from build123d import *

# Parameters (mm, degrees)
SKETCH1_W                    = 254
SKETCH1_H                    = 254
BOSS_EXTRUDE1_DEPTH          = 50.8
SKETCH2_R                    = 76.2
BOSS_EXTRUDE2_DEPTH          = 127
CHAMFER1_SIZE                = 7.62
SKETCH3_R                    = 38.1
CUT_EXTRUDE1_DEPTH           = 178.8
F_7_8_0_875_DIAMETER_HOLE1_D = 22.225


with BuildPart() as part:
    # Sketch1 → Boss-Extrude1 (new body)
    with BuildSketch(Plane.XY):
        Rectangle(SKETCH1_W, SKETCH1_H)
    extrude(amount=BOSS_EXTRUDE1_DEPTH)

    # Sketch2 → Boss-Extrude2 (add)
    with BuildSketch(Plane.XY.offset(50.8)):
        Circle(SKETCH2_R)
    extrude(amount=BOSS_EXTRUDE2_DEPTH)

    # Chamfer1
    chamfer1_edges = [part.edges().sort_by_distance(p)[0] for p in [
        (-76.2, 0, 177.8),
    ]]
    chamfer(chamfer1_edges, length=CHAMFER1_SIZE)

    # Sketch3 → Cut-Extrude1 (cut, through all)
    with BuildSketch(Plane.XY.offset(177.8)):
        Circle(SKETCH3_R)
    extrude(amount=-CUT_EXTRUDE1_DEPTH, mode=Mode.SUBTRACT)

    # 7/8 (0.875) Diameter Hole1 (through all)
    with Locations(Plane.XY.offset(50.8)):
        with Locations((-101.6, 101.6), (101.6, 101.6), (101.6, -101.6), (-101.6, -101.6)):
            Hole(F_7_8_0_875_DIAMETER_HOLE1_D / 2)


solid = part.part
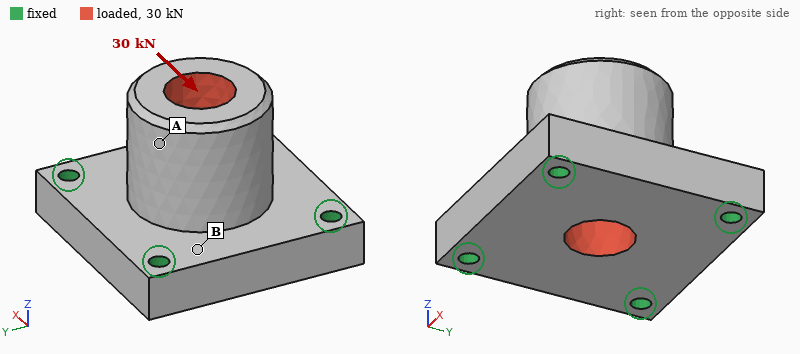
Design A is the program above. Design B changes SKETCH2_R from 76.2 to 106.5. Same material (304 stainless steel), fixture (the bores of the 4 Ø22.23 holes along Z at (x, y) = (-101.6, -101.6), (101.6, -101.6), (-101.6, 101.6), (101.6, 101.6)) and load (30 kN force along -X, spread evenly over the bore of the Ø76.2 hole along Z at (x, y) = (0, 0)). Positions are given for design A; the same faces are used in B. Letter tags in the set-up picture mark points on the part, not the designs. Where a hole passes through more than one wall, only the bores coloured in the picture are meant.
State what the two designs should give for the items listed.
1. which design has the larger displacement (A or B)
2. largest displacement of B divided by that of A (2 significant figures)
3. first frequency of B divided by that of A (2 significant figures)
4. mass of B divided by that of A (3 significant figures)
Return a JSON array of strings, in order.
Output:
["A", "0.44", "1.0", "1.47"]
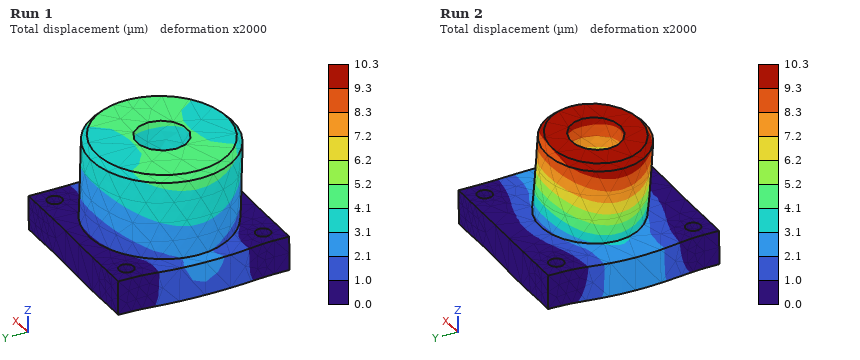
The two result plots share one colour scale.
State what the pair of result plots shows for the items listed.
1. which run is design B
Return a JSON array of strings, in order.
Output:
["Run 1"]
